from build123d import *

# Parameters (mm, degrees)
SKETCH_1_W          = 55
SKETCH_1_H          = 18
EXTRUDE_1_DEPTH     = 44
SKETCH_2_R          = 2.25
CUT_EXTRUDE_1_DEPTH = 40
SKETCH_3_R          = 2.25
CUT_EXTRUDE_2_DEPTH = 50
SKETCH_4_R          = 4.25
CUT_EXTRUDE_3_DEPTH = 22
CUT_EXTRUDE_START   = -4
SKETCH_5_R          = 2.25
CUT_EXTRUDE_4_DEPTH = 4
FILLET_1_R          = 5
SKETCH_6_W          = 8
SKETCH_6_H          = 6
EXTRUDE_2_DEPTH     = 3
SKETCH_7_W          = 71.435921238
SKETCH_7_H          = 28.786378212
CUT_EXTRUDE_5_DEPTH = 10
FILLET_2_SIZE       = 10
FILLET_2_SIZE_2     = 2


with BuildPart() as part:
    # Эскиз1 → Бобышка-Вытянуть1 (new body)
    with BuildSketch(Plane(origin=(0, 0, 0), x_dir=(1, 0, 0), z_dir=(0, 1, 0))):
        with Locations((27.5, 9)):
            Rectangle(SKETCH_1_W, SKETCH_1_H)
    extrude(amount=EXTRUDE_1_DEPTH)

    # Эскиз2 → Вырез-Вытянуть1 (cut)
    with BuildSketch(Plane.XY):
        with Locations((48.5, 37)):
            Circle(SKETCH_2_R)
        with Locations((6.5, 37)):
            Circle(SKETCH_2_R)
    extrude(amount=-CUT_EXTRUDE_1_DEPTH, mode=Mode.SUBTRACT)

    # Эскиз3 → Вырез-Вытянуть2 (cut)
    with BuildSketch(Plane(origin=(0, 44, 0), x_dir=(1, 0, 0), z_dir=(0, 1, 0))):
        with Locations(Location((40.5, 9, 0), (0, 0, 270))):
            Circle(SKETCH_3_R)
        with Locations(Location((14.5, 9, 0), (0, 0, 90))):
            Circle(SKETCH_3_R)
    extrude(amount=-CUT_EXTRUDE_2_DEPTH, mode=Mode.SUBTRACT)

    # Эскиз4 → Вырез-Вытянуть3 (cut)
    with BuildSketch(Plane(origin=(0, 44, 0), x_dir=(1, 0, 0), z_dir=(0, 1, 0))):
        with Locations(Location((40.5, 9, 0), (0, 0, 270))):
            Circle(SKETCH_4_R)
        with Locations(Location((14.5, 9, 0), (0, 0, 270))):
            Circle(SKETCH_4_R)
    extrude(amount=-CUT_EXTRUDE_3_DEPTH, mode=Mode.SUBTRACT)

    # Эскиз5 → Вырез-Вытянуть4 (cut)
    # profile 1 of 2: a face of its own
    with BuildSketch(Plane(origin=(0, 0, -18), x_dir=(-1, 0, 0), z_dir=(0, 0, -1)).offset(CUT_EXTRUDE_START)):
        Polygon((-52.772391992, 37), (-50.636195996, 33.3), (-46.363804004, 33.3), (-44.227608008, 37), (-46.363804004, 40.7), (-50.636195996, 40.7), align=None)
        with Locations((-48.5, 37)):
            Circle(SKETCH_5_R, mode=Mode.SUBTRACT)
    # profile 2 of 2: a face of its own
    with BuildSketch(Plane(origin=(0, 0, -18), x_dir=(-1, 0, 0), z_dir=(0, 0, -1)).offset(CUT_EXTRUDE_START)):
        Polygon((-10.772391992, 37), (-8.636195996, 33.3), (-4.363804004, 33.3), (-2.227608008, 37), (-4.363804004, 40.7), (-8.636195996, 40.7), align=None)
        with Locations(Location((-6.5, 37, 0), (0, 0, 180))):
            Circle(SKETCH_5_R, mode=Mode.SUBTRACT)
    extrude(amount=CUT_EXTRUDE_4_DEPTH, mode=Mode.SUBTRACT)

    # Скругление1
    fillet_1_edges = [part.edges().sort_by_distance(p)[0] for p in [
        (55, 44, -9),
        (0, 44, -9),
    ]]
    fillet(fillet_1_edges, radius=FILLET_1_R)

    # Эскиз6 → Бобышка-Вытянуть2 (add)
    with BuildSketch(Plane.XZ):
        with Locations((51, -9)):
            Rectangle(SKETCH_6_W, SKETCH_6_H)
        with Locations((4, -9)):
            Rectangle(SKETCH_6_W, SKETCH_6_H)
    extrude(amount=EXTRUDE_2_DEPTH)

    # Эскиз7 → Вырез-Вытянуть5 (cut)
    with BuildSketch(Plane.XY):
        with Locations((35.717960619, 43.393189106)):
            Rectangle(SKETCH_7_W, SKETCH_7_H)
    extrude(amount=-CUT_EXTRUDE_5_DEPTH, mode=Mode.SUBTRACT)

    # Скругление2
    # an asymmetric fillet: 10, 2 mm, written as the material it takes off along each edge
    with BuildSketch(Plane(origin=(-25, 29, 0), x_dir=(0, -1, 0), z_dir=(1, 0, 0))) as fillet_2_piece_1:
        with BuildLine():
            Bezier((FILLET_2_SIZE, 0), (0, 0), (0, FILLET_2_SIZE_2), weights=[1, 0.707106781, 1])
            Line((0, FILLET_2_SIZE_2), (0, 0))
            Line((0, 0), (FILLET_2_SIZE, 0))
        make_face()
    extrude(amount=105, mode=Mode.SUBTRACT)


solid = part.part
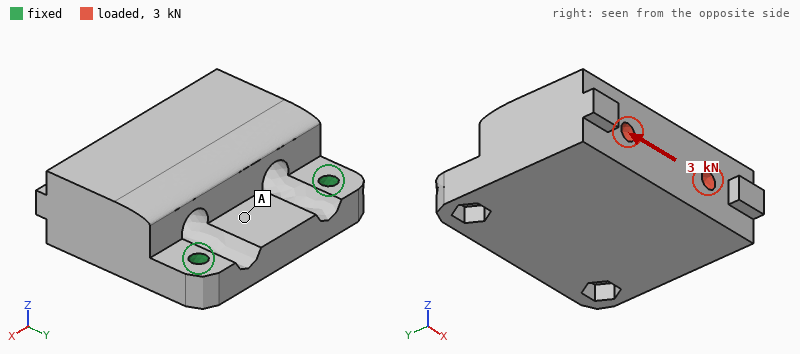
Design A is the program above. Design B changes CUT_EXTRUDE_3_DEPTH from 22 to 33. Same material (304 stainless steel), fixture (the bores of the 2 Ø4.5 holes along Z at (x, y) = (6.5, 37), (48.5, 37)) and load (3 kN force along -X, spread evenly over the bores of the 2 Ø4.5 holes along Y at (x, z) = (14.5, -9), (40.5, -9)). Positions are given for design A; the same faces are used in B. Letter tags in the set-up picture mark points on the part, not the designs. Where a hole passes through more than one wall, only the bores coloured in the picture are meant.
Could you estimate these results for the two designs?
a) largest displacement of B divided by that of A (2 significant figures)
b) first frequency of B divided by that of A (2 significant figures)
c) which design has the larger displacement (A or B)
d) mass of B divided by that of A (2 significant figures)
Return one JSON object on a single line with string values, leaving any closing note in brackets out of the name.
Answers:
{"largest displacement of B divided by that of A": "1.2", "first frequency of B divided by that of A": "1.0", "which design has the larger displacement": "B", "mass of B divided by that of A": "0.97"}
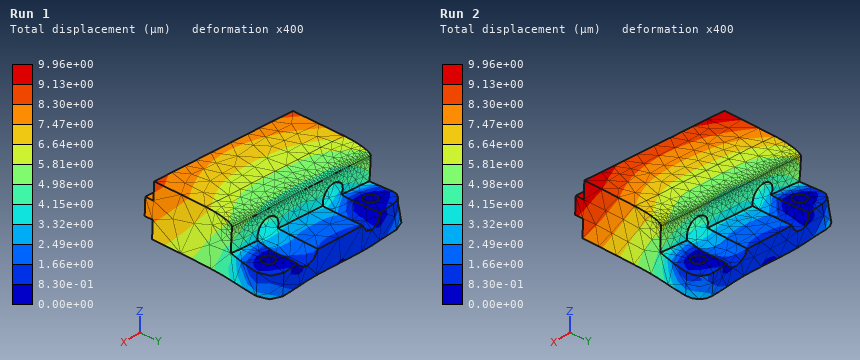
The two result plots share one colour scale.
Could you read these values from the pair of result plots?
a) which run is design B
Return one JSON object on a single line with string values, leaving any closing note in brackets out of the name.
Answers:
{"which run is design B": "Run 2"}
